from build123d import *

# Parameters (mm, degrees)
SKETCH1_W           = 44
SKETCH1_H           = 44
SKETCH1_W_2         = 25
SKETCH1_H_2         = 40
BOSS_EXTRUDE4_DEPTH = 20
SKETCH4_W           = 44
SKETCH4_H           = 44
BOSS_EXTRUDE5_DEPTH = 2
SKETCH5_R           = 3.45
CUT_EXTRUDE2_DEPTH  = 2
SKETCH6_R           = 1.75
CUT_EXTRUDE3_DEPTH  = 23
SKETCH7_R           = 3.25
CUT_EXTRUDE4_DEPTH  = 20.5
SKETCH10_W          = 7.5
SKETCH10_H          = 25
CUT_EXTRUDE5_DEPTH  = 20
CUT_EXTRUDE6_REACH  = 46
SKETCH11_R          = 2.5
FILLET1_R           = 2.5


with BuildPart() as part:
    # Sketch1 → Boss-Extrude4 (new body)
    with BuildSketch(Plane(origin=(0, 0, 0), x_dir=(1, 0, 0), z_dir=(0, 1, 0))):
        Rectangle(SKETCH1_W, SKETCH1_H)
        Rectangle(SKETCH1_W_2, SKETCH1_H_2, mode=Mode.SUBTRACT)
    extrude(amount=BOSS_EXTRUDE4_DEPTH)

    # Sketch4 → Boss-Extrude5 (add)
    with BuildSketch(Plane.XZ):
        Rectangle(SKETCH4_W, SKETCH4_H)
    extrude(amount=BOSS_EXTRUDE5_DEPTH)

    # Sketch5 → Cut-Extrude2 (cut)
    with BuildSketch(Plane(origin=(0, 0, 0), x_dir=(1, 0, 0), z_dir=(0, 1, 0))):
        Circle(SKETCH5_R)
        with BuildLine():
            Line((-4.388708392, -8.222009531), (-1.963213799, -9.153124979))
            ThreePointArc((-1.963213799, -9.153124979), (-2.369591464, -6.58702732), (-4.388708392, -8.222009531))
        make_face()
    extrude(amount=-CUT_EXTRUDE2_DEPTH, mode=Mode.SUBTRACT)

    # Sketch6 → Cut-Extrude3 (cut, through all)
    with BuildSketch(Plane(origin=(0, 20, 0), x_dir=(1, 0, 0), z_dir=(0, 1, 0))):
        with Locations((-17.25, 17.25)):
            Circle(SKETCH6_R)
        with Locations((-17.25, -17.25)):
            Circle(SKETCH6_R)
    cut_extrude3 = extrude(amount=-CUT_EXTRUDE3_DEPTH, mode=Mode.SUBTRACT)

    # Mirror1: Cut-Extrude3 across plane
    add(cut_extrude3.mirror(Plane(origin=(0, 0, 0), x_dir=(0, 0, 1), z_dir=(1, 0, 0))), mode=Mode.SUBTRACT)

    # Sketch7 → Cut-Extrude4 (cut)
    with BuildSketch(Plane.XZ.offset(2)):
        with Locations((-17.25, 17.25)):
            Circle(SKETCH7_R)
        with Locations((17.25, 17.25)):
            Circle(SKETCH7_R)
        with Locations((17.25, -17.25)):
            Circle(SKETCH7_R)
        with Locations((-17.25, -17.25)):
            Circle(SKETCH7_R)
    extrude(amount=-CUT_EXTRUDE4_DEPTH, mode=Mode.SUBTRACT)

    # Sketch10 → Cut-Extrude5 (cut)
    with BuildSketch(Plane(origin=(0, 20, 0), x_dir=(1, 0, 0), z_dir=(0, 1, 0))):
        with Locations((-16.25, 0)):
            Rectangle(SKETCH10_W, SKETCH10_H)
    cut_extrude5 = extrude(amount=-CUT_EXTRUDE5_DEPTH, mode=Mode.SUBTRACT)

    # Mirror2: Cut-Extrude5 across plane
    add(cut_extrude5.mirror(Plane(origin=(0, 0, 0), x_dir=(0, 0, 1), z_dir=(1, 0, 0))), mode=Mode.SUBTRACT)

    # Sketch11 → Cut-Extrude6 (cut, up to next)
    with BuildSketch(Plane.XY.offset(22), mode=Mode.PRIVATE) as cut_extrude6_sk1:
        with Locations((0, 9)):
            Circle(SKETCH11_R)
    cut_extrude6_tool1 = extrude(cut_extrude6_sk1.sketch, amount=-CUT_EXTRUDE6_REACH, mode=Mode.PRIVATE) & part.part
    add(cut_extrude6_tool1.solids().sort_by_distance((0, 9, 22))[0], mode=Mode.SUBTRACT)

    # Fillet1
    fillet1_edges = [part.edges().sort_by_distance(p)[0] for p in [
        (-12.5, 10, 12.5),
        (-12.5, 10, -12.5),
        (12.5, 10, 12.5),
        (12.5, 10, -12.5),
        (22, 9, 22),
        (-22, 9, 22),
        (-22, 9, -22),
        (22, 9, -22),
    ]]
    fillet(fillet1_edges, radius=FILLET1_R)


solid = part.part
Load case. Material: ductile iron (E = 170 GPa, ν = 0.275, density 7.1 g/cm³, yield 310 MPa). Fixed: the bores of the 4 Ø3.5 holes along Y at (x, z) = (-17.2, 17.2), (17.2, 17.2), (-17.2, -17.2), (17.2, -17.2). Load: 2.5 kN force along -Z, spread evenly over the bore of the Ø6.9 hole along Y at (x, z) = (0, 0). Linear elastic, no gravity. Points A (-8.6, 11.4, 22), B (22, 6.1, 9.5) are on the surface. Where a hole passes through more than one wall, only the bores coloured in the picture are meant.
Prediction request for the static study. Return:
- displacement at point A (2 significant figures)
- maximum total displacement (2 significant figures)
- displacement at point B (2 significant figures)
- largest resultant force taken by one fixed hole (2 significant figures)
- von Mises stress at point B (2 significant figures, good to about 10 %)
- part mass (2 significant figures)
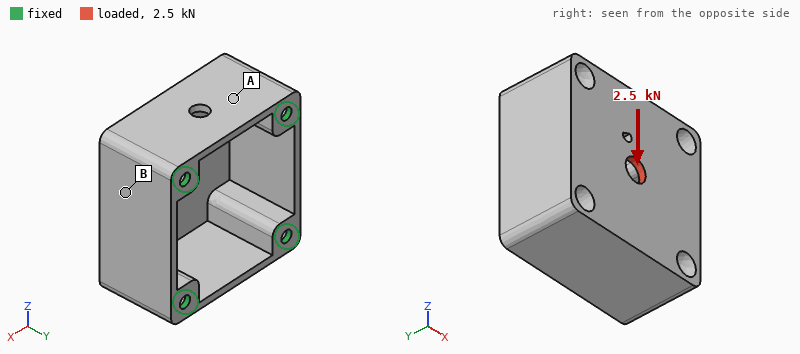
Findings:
6.7 µm
18 µm
7.9 µm
940 N
28 MPa
85 g
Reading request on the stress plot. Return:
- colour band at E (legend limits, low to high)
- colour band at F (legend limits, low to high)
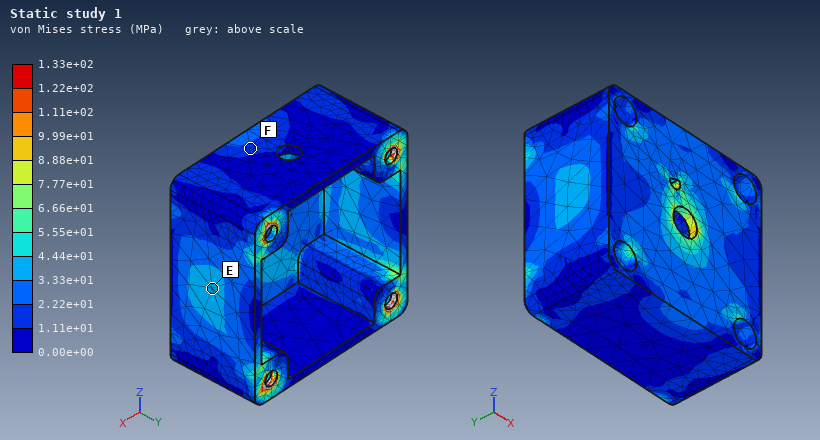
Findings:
3.33e+01 to 4.44e+01 MPa
1.11e+01 to 2.22e+01 MPa
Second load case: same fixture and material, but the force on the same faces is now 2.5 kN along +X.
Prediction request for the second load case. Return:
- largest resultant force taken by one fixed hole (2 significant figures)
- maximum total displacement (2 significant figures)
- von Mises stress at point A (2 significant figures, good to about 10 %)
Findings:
960 N
18 µm
37 MPa
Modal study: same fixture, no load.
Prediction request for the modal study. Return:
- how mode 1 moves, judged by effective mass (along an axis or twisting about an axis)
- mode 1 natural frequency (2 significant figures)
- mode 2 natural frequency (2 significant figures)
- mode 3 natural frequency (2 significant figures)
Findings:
along Y
9000 Hz
10 kHz
10 kHz
